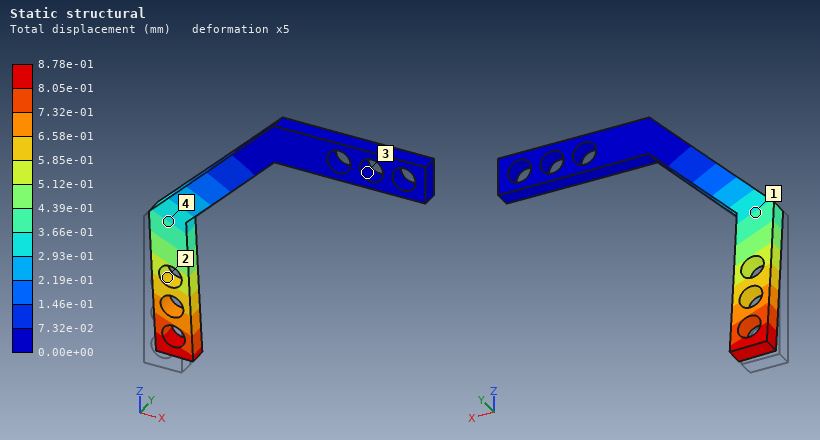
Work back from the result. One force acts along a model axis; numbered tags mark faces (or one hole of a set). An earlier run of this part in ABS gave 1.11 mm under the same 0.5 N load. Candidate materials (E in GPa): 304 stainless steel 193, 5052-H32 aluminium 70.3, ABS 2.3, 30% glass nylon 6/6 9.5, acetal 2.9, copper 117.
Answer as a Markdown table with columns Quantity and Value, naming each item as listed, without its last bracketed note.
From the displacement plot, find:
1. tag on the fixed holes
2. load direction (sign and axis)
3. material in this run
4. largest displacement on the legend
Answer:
| Quantity | Value |
|---|---|
| tag on the fixed holes | 3 |
| load direction | +Y |
| material in this run | acetal |
| largest displacement on the legend | 8.78e-01 mm |
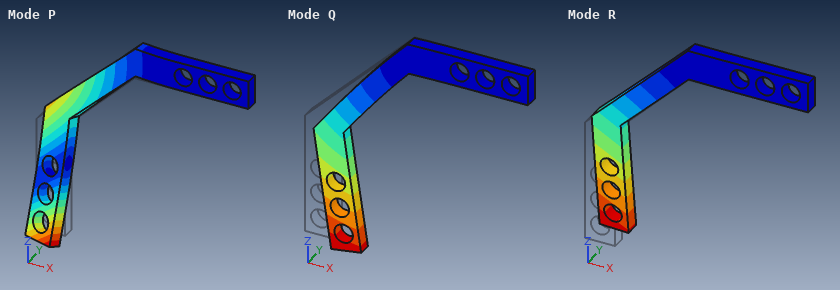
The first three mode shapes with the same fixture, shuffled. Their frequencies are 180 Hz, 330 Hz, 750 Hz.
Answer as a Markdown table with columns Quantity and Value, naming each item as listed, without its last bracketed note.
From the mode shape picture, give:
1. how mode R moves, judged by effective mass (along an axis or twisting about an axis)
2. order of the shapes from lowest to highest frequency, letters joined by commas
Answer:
| Quantity | Value |
|---|---|
| how mode R moves, judged by effective mass | along Y |
| order of the shapes from lowest to highest frequency, letters joined by commas | R, Q, P |
